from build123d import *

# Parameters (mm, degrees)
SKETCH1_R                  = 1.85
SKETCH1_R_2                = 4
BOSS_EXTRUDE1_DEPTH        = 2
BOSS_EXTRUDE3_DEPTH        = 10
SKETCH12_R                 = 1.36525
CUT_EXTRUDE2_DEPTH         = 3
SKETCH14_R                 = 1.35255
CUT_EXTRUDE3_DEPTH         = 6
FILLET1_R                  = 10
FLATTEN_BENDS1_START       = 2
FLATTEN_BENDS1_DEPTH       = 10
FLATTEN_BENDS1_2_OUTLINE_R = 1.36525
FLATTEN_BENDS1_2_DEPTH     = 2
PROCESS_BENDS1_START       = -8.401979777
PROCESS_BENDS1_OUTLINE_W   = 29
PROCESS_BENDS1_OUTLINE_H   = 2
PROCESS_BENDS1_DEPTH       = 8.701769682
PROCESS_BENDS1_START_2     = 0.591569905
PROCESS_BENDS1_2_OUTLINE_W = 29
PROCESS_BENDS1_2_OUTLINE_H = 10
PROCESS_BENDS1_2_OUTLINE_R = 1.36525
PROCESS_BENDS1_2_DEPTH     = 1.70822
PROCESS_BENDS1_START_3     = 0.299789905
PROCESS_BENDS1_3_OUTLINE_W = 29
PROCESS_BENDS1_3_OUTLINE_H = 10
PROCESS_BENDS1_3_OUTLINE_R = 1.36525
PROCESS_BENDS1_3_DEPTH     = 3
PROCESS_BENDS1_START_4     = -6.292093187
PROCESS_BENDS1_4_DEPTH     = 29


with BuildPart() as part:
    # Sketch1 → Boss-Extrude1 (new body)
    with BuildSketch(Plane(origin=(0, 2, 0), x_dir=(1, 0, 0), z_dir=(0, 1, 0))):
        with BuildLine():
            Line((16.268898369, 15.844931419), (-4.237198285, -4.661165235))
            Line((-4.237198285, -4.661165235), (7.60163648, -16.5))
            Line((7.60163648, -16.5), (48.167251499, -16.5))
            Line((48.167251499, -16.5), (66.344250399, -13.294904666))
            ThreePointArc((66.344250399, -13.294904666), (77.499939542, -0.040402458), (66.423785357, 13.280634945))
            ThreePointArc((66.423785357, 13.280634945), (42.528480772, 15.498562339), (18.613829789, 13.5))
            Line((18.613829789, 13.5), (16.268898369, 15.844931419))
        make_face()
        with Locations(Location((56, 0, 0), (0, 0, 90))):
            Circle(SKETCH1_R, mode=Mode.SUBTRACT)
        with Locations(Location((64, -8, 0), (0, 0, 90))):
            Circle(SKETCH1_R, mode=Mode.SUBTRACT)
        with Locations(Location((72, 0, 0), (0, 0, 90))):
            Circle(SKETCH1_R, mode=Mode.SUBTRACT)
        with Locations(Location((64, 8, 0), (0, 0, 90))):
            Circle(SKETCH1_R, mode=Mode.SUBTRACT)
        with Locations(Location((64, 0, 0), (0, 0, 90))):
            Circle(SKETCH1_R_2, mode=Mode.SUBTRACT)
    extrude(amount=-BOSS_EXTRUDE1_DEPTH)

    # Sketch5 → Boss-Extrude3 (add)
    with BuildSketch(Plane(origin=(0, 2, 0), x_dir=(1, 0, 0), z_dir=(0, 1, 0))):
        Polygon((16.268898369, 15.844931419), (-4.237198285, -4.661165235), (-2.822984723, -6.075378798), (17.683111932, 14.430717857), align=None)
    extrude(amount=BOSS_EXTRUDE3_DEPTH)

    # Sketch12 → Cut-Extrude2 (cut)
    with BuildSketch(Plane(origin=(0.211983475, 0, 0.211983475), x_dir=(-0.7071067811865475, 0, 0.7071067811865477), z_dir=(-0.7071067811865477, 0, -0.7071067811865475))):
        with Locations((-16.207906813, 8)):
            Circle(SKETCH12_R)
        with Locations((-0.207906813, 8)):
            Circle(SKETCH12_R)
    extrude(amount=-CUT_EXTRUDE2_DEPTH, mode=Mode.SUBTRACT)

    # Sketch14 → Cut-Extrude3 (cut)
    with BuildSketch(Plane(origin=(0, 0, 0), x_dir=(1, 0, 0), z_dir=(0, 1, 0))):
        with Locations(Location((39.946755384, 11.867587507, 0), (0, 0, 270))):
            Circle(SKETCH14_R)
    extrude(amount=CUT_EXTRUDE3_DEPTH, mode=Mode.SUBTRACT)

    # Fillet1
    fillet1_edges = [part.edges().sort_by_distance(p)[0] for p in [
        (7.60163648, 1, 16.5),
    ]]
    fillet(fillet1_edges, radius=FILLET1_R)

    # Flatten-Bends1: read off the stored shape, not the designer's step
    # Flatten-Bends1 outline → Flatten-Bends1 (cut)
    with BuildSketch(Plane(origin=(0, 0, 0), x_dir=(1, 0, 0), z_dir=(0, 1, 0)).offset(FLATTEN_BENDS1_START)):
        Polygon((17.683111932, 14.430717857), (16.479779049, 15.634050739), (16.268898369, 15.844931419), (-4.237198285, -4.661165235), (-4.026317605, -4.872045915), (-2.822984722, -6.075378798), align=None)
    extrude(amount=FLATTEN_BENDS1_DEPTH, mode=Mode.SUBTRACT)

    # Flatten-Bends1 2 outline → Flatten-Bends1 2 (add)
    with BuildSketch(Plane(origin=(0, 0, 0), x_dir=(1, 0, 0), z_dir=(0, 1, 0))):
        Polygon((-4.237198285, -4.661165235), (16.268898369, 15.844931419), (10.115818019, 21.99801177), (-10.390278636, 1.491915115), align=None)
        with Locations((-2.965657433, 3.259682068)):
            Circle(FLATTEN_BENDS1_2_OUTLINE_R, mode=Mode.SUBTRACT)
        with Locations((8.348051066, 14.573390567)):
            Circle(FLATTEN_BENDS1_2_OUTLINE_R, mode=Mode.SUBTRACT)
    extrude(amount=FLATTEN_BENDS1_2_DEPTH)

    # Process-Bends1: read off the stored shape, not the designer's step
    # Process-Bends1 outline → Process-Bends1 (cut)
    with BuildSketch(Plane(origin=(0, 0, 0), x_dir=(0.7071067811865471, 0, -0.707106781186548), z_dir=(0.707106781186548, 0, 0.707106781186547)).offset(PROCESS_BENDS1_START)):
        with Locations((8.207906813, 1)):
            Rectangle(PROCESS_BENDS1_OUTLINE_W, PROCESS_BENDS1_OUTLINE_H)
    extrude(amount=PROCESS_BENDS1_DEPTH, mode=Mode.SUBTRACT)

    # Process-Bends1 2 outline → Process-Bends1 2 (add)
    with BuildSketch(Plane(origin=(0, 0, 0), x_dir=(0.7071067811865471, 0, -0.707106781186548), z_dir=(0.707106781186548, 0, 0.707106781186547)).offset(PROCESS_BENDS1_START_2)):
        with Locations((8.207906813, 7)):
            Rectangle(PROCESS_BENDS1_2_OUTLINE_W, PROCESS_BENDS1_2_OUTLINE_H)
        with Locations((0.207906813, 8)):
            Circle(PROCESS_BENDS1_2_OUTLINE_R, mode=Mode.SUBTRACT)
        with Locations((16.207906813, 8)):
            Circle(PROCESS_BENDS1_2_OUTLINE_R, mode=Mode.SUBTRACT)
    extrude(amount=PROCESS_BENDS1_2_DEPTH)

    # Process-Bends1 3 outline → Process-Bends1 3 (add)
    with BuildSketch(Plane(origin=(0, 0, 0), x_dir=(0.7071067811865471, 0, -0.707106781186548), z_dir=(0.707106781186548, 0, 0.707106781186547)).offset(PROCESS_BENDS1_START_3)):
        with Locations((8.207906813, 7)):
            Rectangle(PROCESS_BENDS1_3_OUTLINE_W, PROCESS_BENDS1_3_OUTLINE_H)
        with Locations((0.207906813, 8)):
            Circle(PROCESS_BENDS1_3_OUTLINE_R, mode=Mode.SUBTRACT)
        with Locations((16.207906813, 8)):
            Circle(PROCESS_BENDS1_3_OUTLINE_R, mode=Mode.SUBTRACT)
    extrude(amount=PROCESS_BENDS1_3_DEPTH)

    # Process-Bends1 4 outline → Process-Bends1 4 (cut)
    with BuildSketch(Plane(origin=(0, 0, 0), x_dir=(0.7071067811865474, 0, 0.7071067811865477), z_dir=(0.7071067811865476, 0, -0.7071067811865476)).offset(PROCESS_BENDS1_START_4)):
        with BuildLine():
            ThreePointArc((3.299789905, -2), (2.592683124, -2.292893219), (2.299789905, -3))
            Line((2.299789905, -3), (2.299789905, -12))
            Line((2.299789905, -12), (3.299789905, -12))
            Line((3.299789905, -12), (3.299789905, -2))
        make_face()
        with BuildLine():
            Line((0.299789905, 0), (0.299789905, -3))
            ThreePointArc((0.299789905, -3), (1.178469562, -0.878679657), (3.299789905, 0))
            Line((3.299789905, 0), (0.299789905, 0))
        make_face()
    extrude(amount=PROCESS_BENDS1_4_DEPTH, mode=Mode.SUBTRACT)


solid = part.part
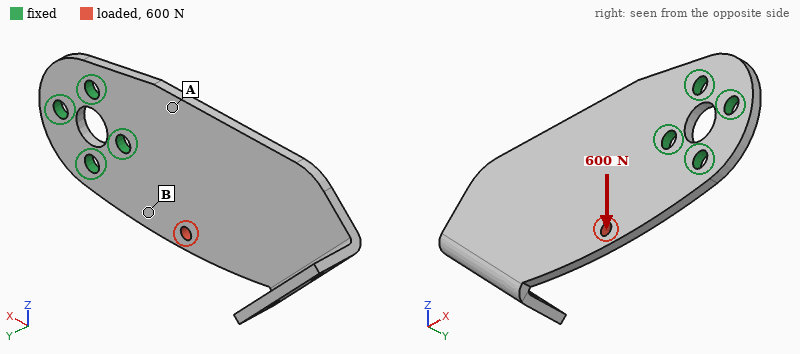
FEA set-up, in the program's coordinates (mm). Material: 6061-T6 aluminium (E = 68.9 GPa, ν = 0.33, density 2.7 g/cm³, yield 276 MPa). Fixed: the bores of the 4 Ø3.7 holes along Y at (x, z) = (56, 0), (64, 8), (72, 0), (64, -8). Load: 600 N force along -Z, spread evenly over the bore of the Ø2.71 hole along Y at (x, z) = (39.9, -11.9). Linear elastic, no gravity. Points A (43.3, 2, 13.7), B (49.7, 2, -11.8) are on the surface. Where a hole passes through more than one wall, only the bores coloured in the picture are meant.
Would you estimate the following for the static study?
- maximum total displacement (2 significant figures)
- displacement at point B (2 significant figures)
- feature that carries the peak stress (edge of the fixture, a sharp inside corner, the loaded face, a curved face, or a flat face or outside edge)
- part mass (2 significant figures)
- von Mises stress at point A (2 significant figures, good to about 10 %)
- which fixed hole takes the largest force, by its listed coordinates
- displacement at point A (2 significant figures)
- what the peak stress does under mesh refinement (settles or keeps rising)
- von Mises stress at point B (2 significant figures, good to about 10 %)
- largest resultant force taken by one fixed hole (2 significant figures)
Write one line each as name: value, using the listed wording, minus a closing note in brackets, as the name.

maximum total displacement: 43 µm
displacement at point B: 9.3 µm
feature that carries the peak stress: edge of the fixture
part mass: 12 g
von Mises stress at point A: 7.8 MPa
which fixed hole takes the largest force, by its listed coordinates: (56, 0)
displacement at point A: 14 µm
what the peak stress does under mesh refinement: keeps rising
von Mises stress at point B: 18 MPa
largest resultant force taken by one fixed hole: 720 N
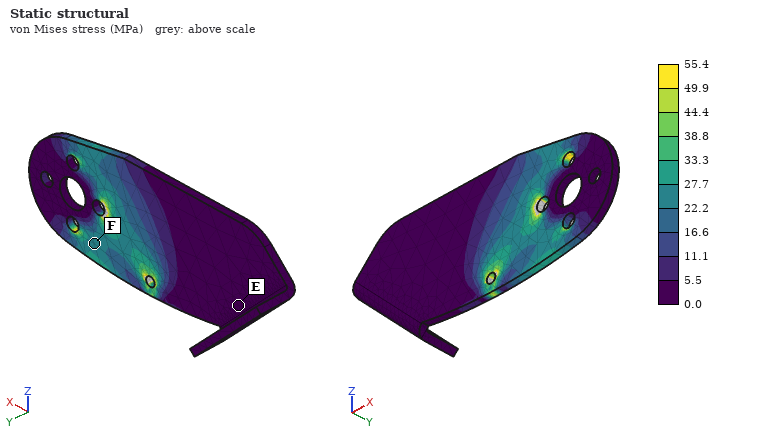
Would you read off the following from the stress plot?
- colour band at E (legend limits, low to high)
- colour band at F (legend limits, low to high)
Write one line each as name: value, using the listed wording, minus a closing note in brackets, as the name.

colour band at E: 0.0 to 5.5 MPa
colour band at F: 22.2 to 27.7 MPa
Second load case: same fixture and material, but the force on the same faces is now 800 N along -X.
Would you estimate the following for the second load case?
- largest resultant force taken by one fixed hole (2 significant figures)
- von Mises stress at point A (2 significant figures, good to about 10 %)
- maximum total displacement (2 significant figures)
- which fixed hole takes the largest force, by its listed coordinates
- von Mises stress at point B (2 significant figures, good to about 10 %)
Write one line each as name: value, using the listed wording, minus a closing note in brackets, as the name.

largest resultant force taken by one fixed hole: 620 N
von Mises stress at point A: 9.0 MPa
maximum total displacement: 43 µm
which fixed hole takes the largest force, by its listed coordinates: (64, -8)
von Mises stress at point B: 37 MPa
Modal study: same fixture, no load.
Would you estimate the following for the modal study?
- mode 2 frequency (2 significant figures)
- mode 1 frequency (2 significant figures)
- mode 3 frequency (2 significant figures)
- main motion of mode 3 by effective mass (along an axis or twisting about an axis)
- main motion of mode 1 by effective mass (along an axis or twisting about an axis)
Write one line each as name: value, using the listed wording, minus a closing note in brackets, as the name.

mode 2 frequency: 1700 Hz
mode 1 frequency: 480 Hz
mode 3 frequency: 2700 Hz
main motion of mode 3 by effective mass: along Y
main motion of mode 1 by effective mass: along Y
